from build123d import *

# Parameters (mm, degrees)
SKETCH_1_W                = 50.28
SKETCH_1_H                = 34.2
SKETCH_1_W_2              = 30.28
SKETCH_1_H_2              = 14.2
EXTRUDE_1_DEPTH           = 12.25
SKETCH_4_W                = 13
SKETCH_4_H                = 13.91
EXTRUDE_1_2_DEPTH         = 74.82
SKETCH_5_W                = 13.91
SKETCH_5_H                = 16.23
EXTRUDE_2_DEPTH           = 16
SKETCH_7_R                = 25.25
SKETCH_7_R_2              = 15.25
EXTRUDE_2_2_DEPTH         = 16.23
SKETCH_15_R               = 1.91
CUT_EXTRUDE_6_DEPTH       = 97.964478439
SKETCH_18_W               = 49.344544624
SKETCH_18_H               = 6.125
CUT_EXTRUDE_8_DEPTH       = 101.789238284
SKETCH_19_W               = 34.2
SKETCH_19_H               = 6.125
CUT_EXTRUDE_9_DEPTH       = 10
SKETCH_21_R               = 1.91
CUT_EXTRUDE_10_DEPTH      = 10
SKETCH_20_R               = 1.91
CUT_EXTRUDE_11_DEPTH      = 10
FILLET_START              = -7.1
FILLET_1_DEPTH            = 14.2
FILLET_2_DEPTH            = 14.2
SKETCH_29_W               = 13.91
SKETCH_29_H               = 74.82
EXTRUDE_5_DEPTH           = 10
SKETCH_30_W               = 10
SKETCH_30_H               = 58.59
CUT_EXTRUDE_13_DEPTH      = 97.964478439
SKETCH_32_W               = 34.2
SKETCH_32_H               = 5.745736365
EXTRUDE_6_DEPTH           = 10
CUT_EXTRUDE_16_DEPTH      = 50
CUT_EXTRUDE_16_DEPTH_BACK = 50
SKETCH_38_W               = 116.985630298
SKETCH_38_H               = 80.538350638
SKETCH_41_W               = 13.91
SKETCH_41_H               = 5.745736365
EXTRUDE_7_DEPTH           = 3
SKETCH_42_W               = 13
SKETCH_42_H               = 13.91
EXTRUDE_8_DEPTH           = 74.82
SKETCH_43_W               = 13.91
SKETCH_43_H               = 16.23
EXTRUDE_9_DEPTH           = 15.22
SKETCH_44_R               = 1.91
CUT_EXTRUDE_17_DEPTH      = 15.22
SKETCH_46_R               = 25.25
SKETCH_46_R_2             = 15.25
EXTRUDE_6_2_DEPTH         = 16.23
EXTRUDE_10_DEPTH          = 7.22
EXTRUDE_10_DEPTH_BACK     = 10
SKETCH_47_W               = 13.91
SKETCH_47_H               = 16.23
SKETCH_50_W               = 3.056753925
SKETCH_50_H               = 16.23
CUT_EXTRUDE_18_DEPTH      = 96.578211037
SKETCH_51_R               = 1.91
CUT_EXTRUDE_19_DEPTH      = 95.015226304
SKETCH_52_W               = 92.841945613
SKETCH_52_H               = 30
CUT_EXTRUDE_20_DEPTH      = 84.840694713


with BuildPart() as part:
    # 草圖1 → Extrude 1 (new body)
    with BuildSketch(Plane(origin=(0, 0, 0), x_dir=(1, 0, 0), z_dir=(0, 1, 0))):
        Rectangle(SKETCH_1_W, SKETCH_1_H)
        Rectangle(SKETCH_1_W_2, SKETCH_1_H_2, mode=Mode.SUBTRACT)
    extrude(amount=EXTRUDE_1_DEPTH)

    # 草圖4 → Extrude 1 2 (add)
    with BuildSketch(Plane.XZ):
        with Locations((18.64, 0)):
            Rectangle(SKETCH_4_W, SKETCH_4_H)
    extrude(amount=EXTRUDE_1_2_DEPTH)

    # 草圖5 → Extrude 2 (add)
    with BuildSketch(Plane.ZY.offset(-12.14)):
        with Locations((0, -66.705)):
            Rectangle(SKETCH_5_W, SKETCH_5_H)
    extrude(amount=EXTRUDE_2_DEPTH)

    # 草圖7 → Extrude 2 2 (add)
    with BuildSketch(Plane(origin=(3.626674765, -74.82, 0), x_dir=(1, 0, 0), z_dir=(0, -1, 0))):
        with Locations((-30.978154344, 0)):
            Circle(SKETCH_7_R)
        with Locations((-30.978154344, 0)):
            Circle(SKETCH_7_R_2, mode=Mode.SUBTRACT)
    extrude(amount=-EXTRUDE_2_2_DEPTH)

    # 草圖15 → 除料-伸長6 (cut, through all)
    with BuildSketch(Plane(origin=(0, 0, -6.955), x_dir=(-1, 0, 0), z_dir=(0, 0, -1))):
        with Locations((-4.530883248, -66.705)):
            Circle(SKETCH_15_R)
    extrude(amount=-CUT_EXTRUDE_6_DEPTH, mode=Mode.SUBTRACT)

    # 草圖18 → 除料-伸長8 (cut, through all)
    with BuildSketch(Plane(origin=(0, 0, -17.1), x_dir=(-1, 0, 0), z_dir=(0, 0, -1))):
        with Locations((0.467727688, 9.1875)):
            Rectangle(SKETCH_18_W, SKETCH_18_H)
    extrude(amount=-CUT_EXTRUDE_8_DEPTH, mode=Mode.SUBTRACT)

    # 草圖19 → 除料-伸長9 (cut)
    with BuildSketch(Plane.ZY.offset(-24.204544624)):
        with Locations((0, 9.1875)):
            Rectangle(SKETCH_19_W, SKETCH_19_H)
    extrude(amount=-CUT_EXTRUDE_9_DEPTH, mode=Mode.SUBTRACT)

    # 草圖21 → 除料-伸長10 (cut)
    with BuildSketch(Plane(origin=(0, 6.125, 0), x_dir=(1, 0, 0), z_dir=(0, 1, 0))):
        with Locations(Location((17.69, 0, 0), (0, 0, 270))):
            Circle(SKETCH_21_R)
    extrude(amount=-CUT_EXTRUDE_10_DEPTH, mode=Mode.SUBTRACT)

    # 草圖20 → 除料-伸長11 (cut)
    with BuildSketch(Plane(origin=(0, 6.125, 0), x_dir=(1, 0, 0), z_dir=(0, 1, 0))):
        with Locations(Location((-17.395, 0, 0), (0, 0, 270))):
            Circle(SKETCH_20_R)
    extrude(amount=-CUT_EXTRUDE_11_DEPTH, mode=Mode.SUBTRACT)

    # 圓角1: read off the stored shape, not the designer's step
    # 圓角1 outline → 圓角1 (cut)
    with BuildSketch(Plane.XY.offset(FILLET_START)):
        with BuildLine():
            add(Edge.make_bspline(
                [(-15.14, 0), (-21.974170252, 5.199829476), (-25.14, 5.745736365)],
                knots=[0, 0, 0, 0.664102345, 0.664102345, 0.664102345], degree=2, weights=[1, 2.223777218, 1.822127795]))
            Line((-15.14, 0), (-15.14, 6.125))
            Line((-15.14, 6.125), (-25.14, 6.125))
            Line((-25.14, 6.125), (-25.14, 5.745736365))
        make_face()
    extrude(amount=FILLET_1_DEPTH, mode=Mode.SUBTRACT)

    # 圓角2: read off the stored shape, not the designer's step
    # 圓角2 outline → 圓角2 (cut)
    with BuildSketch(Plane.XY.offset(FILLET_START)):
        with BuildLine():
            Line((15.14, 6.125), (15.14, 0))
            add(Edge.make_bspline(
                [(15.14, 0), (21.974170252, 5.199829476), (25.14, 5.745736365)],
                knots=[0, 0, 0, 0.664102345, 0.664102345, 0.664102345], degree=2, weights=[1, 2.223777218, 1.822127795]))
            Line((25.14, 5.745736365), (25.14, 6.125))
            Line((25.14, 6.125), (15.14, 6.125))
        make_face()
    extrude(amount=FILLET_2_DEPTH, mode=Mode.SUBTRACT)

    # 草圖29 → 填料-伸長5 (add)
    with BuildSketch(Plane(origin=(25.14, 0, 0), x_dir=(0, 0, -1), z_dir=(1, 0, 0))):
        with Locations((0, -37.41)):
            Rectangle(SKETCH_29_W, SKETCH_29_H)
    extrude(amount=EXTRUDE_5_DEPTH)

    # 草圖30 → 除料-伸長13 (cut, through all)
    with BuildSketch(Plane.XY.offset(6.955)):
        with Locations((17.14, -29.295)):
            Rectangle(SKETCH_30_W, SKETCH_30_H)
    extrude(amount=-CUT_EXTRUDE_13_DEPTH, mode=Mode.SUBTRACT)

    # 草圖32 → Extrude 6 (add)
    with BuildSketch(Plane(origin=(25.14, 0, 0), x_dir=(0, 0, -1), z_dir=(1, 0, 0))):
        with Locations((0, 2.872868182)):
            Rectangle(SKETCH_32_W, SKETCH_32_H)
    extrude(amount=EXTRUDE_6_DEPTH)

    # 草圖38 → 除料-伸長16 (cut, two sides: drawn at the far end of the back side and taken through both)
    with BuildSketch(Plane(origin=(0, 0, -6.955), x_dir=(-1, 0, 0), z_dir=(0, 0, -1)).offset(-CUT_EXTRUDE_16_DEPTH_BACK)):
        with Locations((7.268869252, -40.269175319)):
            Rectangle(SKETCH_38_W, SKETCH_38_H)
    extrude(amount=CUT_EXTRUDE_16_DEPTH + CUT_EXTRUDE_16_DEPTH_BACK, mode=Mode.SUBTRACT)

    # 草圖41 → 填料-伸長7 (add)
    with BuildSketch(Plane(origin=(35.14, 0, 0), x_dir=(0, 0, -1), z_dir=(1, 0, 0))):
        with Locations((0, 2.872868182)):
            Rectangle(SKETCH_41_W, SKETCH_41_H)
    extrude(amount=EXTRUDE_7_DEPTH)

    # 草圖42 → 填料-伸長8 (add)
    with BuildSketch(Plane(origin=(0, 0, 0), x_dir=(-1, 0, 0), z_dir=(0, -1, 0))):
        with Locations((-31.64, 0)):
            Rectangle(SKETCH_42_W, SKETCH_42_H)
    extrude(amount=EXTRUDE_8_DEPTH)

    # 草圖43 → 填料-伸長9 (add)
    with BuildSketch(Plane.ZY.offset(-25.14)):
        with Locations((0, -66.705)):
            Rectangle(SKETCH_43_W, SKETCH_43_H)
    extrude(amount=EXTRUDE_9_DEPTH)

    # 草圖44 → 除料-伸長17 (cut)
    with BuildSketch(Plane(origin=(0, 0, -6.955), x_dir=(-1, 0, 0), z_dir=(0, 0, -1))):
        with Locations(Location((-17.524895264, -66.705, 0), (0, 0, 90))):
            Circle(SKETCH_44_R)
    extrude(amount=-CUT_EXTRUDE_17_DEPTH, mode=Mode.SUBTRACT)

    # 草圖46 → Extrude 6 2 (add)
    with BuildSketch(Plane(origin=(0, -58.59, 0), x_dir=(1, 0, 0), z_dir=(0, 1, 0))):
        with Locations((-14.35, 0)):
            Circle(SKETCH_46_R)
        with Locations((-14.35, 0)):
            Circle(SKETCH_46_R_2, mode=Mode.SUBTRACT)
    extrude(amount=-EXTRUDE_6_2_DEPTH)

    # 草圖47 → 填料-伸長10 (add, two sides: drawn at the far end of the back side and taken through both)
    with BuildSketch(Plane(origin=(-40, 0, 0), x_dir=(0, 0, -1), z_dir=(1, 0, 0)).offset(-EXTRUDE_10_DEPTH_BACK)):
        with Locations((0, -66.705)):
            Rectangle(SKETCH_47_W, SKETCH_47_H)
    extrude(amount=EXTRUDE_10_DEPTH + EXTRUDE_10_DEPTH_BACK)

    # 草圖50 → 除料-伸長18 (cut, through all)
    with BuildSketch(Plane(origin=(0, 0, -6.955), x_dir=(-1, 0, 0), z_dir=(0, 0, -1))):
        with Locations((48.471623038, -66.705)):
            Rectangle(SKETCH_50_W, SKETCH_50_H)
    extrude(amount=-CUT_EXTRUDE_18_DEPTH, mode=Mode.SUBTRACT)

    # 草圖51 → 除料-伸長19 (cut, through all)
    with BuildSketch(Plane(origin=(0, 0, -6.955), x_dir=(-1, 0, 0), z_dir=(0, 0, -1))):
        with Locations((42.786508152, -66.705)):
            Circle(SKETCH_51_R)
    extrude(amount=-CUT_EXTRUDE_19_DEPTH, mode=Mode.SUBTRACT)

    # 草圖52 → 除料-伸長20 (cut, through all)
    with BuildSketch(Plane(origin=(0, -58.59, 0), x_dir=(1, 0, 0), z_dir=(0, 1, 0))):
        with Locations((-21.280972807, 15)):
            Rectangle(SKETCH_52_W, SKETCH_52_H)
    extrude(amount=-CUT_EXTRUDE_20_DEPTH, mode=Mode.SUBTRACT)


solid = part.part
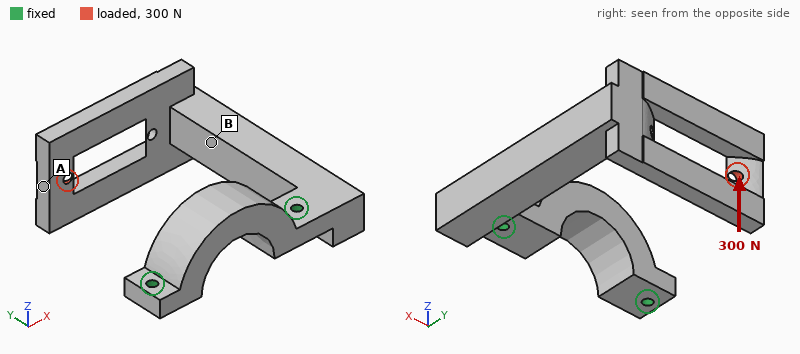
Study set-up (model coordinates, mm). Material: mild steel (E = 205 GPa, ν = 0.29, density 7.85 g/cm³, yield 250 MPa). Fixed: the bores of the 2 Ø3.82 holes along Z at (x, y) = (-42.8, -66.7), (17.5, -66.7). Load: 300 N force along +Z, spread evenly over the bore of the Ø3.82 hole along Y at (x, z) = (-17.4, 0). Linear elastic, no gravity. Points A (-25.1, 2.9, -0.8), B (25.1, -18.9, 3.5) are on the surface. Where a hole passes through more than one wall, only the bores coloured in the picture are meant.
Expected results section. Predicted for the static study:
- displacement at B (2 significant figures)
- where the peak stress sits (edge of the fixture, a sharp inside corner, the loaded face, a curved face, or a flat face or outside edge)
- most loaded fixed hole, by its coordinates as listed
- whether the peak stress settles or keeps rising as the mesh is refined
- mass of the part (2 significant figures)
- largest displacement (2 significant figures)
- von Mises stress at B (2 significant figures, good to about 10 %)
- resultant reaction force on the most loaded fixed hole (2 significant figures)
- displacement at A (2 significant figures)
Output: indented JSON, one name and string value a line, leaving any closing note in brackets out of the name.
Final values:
{
  "displacement at B": "0.11 mm",
  "where the peak stress sits": "edge of the fixture",
  "most loaded fixed hole, by its coordinates as listed": "(17.5, -66.7)",
  "whether the peak stress settles or keeps rising as the mesh is refined": "keeps rising",
  "mass of the part": "280 g",
  "largest displacement": "0.42 mm",
  "von Mises stress at B": "43 MPa",
  "resultant reaction force on the most loaded fixed hole": "280 N",
  "displacement at A": "0.40 mm"
}
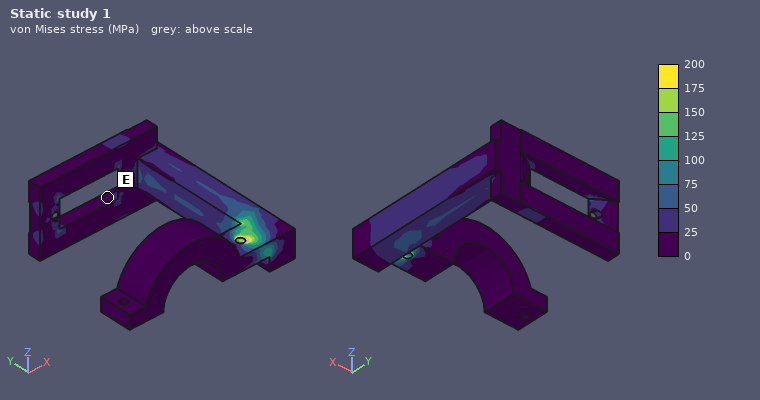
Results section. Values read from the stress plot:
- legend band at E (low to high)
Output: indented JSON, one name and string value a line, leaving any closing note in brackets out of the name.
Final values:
{
  "legend band at E": "0 to 25 MPa"
}
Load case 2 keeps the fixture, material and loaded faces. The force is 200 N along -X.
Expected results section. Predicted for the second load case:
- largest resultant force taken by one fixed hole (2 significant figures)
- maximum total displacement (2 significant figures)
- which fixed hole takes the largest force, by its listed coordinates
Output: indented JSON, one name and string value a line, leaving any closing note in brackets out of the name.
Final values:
{
  "largest resultant force taken by one fixed hole": "230 N",
  "maximum total displacement": "0.11 mm",
  "which fixed hole takes the largest force, by its listed coordinates": "(17.5, -66.7)"
}
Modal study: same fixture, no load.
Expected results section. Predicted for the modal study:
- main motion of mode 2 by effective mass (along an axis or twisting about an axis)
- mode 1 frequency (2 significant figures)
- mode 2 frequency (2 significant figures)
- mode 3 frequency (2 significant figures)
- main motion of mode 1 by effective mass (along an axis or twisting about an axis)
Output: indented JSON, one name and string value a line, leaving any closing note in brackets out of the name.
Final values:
{
  "main motion of mode 2 by effective mass": "along X",
  "mode 1 frequency": "610 Hz",
  "mode 2 frequency": "710 Hz",
  "mode 3 frequency": "1300 Hz",
  "main motion of mode 1 by effective mass": "along Z"
}
